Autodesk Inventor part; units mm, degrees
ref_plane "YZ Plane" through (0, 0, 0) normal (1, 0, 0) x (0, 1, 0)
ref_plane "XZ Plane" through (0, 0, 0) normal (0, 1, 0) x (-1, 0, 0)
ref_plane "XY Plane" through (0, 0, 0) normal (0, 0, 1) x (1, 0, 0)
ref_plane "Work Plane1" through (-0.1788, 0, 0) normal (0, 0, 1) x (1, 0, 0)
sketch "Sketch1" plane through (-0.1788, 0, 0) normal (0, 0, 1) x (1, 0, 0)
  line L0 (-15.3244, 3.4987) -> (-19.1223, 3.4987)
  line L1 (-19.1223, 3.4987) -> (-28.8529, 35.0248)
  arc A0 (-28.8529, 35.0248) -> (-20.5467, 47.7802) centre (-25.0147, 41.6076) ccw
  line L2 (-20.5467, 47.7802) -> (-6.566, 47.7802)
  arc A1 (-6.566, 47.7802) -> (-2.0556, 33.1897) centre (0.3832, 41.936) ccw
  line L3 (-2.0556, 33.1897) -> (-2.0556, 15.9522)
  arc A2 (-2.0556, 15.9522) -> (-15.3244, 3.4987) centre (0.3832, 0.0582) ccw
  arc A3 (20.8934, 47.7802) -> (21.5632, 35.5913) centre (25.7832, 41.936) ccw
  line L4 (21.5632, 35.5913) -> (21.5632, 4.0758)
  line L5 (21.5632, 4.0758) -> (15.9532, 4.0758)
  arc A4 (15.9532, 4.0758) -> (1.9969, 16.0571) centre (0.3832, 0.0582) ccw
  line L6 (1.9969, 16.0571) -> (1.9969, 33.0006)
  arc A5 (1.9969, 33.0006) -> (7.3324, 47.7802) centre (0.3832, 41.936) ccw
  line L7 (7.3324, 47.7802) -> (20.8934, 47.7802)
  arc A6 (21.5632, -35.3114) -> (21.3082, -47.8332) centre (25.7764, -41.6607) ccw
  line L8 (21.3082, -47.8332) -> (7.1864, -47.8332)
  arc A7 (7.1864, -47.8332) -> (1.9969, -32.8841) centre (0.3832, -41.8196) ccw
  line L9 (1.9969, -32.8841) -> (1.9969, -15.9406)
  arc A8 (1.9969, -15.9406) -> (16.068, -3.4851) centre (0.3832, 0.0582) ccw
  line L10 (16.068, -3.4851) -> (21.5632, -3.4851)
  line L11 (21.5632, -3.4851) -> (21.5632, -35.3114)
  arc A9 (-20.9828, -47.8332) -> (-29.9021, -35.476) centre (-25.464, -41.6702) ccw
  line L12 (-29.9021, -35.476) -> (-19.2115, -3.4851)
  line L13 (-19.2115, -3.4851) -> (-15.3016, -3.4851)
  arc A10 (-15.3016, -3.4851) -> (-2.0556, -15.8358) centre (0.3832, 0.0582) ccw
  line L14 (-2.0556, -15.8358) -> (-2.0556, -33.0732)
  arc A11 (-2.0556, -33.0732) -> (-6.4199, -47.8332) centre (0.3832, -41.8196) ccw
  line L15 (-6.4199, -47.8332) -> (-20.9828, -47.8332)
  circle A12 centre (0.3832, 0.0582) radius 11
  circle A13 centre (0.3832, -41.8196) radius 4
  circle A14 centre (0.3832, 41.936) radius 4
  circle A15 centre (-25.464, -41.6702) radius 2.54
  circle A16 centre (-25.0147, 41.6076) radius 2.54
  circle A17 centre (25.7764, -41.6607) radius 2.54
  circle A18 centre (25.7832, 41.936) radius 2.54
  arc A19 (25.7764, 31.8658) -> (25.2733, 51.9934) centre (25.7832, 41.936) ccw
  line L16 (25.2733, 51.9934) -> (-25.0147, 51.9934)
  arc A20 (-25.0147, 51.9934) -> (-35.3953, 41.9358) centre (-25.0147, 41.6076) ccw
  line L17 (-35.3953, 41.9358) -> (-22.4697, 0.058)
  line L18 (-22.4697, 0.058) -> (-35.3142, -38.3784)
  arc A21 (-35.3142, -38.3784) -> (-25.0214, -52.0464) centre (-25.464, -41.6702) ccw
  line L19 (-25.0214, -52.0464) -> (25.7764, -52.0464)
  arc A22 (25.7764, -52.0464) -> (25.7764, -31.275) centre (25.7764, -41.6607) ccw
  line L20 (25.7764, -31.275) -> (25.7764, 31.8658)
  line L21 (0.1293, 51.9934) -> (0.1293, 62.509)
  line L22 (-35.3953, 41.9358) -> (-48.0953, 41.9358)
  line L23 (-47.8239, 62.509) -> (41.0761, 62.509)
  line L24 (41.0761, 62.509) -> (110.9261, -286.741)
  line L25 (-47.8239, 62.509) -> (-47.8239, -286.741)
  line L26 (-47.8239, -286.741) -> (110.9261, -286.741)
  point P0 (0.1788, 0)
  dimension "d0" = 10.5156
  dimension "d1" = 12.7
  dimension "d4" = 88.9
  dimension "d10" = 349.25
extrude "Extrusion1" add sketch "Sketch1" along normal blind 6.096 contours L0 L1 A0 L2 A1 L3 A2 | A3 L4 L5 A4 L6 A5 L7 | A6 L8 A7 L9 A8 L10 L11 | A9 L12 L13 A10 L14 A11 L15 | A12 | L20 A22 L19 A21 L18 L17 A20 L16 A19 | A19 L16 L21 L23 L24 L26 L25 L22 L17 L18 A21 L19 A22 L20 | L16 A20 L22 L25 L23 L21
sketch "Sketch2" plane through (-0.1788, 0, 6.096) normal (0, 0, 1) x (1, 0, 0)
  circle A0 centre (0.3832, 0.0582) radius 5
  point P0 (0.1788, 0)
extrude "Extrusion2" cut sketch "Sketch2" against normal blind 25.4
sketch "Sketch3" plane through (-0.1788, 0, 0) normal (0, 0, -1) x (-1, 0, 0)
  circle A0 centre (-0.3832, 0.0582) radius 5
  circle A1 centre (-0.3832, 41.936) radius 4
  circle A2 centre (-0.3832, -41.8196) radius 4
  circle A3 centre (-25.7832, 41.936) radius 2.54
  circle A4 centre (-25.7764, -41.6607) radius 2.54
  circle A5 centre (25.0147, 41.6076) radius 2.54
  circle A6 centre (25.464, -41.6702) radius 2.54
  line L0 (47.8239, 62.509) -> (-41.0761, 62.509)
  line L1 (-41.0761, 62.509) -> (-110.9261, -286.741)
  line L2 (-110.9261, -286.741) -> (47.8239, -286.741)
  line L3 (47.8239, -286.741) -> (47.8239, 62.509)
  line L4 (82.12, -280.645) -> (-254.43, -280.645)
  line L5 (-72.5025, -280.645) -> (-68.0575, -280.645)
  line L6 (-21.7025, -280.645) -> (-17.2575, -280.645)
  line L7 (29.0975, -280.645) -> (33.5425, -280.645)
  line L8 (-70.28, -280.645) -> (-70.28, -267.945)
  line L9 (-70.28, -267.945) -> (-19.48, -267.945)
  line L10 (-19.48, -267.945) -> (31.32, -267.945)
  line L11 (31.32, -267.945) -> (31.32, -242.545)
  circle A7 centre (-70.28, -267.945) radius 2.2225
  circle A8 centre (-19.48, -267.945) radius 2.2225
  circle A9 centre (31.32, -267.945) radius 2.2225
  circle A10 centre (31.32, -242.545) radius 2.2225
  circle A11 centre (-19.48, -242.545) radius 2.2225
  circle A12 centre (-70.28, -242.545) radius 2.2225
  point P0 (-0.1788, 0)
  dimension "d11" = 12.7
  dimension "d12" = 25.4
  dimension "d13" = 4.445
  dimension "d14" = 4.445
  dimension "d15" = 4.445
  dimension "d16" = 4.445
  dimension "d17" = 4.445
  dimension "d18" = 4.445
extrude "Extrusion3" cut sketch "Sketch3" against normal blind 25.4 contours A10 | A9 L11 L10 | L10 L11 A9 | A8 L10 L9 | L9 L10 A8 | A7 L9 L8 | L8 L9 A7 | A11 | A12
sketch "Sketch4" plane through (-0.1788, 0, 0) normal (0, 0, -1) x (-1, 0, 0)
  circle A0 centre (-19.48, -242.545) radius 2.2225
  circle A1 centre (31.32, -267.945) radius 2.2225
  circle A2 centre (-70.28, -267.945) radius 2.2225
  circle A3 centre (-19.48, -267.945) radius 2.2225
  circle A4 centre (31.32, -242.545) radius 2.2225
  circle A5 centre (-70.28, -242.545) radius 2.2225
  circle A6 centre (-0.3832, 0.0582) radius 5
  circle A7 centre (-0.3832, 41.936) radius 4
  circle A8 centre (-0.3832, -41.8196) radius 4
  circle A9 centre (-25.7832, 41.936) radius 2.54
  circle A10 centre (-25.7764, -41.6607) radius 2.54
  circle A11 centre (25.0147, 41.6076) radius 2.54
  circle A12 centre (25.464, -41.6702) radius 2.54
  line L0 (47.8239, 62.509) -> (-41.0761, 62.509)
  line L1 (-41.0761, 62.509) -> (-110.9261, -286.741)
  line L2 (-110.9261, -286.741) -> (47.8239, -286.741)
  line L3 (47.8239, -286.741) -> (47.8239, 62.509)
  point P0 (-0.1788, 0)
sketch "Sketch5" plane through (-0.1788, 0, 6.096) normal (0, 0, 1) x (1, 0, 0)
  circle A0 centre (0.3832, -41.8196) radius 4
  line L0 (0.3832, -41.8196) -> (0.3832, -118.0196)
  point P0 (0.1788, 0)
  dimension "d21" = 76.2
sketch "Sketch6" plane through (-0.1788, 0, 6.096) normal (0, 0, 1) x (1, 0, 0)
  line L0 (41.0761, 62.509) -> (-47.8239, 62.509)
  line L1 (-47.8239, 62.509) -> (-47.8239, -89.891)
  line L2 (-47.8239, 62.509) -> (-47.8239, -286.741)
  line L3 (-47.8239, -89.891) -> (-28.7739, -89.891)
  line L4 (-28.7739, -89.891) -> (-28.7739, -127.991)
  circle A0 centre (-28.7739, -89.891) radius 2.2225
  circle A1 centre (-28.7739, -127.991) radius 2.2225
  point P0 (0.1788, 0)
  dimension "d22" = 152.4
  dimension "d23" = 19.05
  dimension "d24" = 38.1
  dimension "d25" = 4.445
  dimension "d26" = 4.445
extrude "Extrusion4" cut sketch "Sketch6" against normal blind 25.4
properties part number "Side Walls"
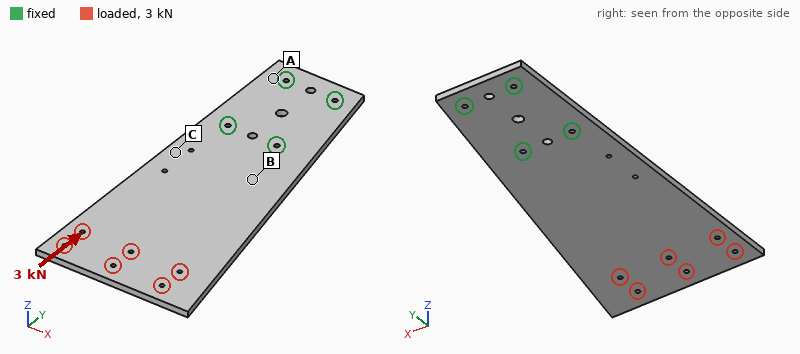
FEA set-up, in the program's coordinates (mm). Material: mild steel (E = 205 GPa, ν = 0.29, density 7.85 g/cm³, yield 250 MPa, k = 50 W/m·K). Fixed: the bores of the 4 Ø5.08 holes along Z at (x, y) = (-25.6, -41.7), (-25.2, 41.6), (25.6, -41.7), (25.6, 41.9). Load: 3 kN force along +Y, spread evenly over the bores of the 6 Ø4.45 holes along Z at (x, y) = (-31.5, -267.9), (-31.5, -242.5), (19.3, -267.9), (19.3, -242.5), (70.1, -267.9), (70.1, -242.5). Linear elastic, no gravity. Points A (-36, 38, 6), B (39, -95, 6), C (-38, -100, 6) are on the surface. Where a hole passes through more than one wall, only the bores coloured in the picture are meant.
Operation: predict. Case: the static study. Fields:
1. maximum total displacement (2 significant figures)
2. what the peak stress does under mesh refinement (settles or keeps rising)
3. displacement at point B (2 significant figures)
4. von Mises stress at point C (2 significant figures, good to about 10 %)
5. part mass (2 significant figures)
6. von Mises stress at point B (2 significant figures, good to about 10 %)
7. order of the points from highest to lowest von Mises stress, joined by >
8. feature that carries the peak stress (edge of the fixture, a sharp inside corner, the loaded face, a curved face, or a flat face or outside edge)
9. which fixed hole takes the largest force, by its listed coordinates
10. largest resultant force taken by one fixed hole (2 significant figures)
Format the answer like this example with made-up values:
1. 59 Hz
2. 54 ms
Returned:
1. 9.5 µm
2. keeps rising
3. 2.8 µm
4. 2.7 MPa
5. 2.1 kg
6. 5.1 MPa
7. B > C > A
8. edge of the fixture
9. (25.6, -41.7)
10. 1.8 kN
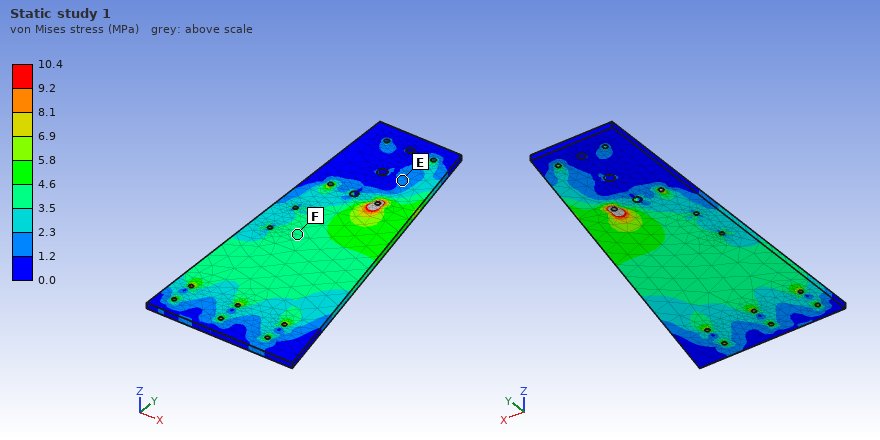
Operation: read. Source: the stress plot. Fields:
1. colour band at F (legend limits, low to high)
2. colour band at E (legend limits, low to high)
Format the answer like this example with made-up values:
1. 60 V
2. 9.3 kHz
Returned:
1. 3.5 to 4.6 MPa
2. 1.2 to 2.3 MPa
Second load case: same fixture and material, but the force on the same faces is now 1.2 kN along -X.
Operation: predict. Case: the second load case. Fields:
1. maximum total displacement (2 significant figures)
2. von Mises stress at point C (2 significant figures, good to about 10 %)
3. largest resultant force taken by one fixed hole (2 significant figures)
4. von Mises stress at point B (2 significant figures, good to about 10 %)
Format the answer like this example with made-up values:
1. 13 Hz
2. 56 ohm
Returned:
1. 52 µm
2. 12 MPa
3. 3.2 kN
4. 7.2 MPa
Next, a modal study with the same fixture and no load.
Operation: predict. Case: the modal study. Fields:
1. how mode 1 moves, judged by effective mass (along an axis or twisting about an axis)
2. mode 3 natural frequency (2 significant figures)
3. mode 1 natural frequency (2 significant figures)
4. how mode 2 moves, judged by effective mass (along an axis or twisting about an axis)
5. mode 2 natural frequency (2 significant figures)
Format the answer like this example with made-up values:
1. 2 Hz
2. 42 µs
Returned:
1. along Z
2. 490 Hz
3. 72 Hz
4. twisting about Y
5. 270 Hz
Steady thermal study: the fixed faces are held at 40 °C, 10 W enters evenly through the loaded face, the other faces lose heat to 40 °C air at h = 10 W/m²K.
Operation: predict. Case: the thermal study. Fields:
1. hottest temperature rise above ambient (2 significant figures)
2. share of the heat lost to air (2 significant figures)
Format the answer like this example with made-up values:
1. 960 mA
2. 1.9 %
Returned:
1. 23 K
2. 79 %
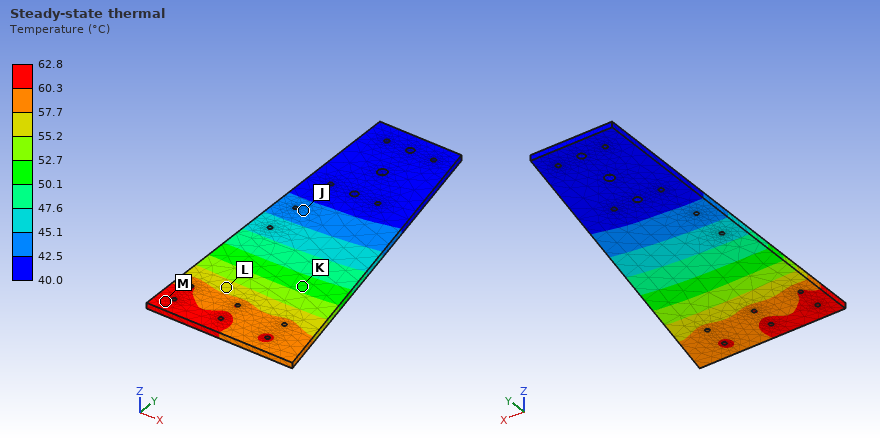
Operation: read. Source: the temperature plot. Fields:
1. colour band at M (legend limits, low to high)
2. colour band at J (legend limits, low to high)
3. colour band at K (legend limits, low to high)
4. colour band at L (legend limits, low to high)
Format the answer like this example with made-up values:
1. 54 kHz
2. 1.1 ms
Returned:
1. 60.3 to 62.8 °C
2. 42.5 to 45.1 °C
3. 50.1 to 52.7 °C
4. 55.2 to 57.7 °C
